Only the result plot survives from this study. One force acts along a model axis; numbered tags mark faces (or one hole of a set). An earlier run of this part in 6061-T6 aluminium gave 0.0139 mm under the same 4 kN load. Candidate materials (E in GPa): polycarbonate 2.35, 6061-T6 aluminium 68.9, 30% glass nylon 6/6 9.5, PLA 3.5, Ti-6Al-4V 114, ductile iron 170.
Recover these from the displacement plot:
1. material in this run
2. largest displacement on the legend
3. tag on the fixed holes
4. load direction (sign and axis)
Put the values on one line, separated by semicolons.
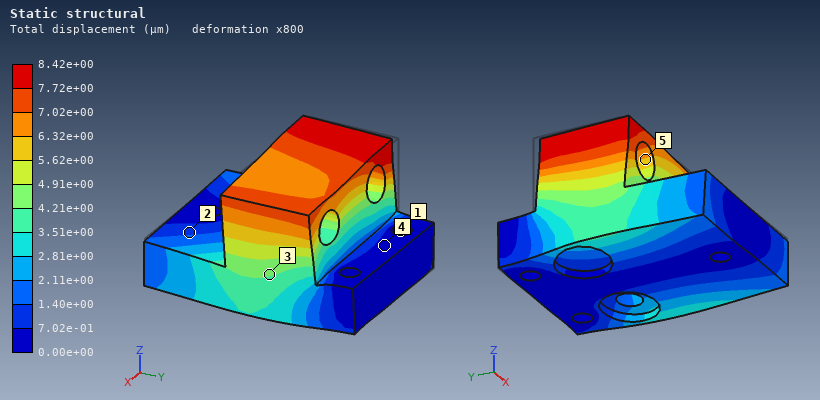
Ti-6Al-4V; 8.42e+00 µm; 1; +X
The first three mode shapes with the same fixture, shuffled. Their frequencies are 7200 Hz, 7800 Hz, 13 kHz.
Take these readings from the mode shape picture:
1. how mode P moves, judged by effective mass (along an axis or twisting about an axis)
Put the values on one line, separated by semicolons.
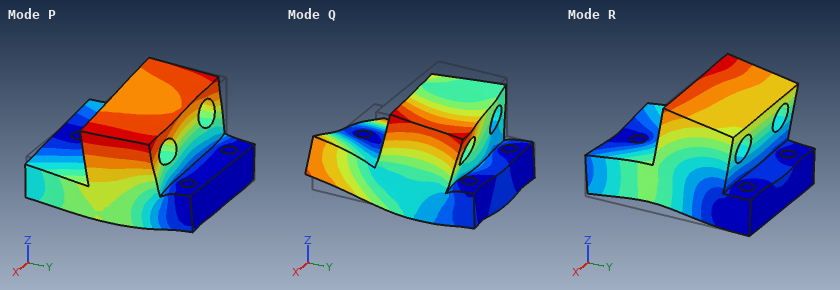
along X
